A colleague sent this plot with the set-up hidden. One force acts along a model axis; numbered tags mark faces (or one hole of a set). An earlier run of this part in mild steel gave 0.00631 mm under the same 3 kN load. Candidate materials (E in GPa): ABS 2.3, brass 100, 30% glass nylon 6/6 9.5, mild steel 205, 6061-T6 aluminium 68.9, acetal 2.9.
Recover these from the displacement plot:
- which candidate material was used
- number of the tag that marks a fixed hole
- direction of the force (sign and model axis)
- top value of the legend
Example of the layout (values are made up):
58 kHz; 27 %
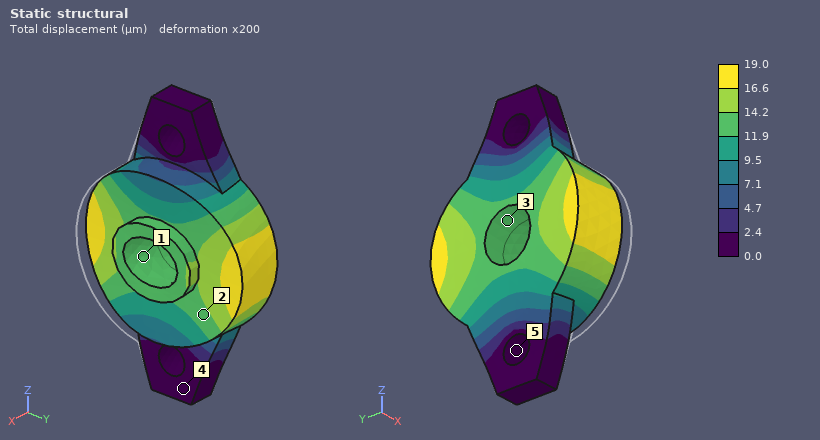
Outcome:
6061-T6 aluminium; 5; -X; 19.0 µm
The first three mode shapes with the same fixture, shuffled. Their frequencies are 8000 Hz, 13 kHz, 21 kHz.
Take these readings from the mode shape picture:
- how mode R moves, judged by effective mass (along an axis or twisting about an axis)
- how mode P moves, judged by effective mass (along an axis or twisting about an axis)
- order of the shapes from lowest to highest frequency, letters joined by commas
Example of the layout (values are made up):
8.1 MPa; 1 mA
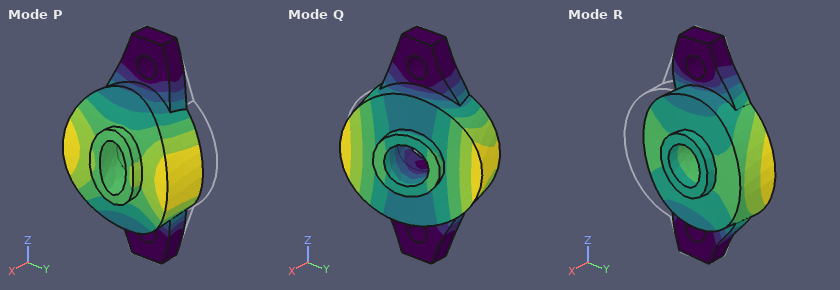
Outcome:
along Y; along X; Q, P, R
